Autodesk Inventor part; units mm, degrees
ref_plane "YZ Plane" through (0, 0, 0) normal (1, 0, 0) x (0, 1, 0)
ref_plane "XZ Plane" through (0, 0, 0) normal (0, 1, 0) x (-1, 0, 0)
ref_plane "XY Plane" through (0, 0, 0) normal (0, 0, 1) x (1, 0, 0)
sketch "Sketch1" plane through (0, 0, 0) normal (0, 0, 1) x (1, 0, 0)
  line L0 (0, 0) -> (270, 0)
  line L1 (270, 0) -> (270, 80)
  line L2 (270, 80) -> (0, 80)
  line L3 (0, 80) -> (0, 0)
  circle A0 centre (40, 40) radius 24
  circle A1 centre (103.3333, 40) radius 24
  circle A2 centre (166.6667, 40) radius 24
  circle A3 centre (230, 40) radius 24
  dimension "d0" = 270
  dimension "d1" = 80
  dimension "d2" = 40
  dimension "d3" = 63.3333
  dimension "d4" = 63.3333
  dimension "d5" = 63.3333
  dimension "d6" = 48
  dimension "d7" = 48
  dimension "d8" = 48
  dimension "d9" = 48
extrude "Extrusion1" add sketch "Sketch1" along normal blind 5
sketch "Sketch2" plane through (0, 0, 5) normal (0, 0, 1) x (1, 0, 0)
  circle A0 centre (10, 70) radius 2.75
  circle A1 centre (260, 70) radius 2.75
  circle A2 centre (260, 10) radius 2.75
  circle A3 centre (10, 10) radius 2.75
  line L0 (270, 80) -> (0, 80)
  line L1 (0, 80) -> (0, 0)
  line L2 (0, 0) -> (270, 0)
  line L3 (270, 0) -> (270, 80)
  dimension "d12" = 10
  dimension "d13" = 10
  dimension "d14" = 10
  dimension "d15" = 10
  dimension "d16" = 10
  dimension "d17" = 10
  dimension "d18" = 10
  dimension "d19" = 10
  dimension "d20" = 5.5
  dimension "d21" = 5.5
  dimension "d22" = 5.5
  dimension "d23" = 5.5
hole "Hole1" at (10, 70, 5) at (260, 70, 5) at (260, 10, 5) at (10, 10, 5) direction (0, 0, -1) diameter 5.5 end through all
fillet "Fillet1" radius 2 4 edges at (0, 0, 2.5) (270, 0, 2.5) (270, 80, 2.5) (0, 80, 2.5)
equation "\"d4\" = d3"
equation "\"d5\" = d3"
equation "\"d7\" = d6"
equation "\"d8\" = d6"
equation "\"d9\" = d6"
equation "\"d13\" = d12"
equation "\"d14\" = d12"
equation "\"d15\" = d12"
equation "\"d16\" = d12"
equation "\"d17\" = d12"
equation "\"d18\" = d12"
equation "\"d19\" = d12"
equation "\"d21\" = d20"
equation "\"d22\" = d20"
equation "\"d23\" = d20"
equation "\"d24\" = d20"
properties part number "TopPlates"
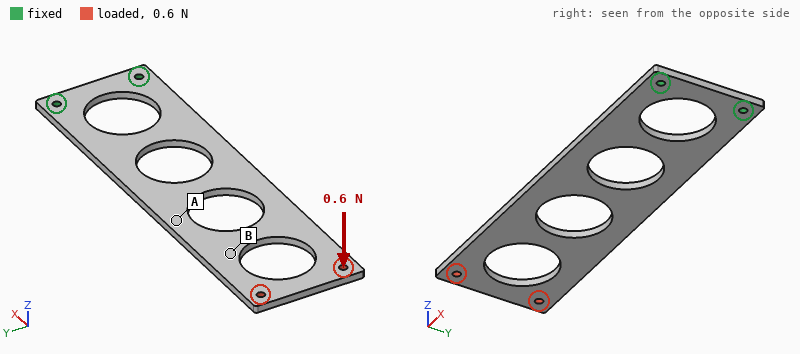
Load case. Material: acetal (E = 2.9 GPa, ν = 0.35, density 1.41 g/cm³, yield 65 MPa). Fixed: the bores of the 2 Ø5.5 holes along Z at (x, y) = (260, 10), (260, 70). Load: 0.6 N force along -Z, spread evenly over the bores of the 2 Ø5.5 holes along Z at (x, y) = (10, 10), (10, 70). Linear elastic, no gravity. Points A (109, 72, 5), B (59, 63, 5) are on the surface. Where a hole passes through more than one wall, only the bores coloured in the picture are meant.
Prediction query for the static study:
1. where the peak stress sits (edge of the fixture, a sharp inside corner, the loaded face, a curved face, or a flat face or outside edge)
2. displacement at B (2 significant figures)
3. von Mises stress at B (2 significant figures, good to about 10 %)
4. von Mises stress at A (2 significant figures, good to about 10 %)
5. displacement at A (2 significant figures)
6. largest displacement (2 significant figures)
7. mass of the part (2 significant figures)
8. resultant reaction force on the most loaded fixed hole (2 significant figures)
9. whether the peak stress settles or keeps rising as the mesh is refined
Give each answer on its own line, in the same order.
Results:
edge of the fixture
1.8 mm
0.16 MPa
0.42 MPa
1.1 mm
2.7 mm
100 g
0.30 N
keeps rising
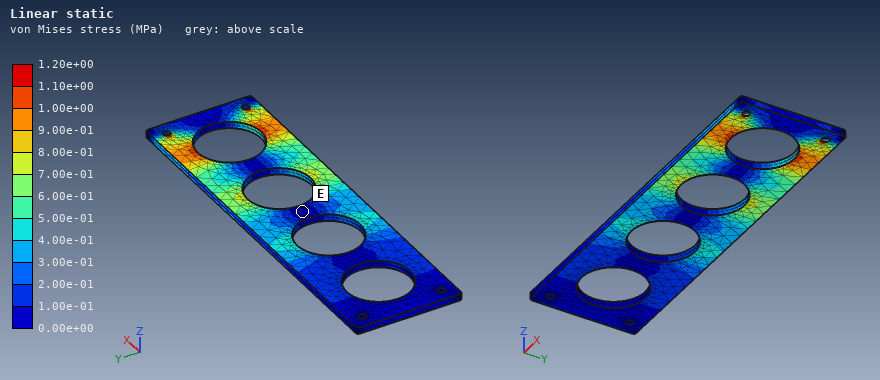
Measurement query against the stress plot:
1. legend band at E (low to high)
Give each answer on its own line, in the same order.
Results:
0.00e+00 to 1.00e-01 MPa
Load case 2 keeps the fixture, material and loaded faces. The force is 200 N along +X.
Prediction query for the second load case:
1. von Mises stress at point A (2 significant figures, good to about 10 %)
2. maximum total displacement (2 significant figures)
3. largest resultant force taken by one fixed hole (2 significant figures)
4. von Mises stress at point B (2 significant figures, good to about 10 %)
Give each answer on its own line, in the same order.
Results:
1.1 MPa
99 µm
100 N
0.72 MPa
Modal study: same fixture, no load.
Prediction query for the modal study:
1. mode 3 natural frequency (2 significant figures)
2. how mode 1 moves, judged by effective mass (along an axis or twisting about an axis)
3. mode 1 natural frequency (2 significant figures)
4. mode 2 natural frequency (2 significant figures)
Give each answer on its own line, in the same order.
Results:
93 Hz
along Z
15 Hz
90 Hz
